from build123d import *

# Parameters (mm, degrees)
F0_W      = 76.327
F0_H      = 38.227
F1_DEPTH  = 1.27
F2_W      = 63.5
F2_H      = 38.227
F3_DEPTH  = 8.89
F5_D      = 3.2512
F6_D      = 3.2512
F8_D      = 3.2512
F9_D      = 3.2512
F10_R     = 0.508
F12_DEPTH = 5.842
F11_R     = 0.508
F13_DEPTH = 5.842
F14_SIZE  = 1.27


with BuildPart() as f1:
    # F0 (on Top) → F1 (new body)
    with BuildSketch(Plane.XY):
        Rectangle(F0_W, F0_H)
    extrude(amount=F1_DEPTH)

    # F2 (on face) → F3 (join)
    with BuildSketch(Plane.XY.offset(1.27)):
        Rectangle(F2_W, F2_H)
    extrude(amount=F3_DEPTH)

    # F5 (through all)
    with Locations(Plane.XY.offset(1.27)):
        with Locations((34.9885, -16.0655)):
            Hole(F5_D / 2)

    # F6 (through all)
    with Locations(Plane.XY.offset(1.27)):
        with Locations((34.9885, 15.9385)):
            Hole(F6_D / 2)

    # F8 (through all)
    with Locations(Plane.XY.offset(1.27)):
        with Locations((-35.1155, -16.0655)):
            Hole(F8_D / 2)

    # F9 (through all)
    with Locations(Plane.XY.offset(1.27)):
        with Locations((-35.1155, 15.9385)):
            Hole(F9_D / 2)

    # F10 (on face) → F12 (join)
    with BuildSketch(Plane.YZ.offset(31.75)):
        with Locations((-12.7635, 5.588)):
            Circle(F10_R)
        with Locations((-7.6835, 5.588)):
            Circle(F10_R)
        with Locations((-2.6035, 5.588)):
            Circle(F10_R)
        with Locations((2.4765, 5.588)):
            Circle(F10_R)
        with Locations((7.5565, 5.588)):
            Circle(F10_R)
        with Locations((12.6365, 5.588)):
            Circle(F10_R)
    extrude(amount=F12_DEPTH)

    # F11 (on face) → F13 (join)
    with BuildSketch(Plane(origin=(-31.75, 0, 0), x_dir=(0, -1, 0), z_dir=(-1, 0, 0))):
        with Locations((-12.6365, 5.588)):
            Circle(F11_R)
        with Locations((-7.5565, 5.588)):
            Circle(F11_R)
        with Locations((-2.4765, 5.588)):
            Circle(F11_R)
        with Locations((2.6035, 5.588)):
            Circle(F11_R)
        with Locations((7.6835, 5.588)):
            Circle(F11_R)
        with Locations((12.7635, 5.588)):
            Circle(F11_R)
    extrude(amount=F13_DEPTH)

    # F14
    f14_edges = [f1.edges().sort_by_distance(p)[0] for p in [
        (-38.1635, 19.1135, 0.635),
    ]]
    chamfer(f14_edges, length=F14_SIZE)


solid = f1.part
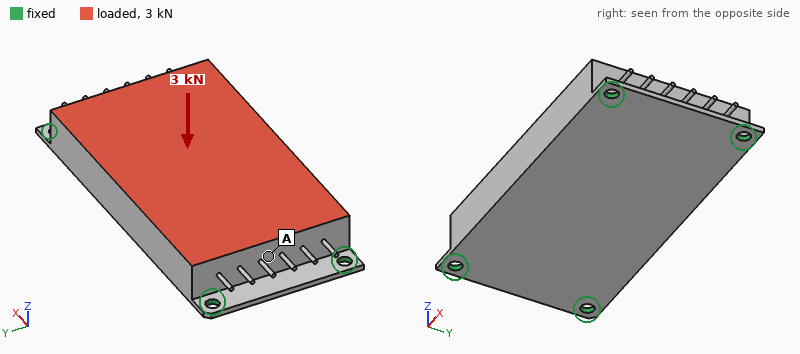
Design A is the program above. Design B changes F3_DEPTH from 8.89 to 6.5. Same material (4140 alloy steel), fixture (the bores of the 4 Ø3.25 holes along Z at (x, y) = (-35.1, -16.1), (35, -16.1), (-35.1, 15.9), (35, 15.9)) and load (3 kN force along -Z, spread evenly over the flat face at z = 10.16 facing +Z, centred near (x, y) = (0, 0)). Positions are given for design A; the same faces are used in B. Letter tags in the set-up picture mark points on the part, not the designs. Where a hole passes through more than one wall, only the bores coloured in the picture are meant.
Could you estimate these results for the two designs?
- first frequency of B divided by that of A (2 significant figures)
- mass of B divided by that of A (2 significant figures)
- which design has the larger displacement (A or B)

0.91
0.77
B
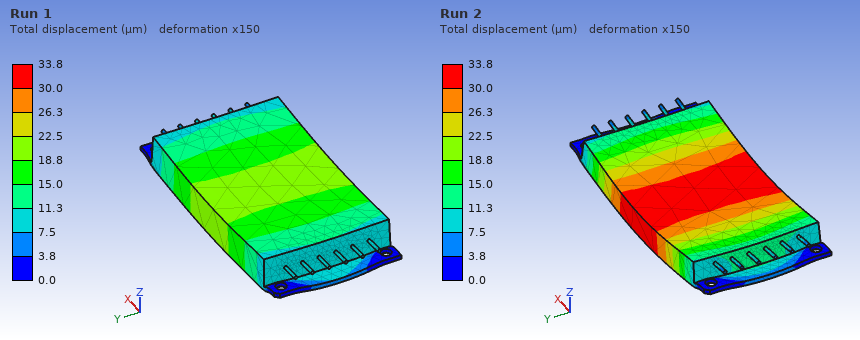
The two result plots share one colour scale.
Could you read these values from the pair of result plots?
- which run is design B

Run 2
